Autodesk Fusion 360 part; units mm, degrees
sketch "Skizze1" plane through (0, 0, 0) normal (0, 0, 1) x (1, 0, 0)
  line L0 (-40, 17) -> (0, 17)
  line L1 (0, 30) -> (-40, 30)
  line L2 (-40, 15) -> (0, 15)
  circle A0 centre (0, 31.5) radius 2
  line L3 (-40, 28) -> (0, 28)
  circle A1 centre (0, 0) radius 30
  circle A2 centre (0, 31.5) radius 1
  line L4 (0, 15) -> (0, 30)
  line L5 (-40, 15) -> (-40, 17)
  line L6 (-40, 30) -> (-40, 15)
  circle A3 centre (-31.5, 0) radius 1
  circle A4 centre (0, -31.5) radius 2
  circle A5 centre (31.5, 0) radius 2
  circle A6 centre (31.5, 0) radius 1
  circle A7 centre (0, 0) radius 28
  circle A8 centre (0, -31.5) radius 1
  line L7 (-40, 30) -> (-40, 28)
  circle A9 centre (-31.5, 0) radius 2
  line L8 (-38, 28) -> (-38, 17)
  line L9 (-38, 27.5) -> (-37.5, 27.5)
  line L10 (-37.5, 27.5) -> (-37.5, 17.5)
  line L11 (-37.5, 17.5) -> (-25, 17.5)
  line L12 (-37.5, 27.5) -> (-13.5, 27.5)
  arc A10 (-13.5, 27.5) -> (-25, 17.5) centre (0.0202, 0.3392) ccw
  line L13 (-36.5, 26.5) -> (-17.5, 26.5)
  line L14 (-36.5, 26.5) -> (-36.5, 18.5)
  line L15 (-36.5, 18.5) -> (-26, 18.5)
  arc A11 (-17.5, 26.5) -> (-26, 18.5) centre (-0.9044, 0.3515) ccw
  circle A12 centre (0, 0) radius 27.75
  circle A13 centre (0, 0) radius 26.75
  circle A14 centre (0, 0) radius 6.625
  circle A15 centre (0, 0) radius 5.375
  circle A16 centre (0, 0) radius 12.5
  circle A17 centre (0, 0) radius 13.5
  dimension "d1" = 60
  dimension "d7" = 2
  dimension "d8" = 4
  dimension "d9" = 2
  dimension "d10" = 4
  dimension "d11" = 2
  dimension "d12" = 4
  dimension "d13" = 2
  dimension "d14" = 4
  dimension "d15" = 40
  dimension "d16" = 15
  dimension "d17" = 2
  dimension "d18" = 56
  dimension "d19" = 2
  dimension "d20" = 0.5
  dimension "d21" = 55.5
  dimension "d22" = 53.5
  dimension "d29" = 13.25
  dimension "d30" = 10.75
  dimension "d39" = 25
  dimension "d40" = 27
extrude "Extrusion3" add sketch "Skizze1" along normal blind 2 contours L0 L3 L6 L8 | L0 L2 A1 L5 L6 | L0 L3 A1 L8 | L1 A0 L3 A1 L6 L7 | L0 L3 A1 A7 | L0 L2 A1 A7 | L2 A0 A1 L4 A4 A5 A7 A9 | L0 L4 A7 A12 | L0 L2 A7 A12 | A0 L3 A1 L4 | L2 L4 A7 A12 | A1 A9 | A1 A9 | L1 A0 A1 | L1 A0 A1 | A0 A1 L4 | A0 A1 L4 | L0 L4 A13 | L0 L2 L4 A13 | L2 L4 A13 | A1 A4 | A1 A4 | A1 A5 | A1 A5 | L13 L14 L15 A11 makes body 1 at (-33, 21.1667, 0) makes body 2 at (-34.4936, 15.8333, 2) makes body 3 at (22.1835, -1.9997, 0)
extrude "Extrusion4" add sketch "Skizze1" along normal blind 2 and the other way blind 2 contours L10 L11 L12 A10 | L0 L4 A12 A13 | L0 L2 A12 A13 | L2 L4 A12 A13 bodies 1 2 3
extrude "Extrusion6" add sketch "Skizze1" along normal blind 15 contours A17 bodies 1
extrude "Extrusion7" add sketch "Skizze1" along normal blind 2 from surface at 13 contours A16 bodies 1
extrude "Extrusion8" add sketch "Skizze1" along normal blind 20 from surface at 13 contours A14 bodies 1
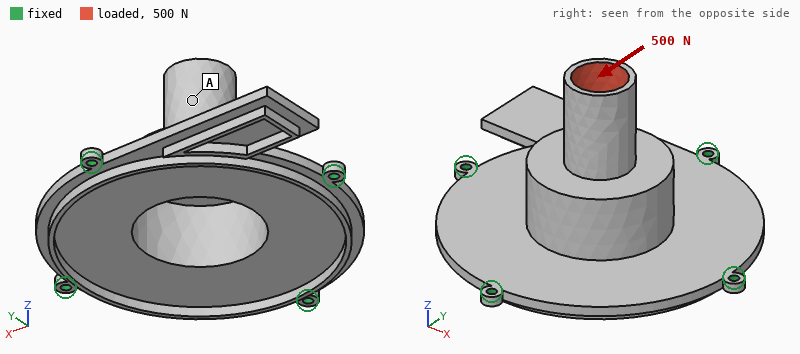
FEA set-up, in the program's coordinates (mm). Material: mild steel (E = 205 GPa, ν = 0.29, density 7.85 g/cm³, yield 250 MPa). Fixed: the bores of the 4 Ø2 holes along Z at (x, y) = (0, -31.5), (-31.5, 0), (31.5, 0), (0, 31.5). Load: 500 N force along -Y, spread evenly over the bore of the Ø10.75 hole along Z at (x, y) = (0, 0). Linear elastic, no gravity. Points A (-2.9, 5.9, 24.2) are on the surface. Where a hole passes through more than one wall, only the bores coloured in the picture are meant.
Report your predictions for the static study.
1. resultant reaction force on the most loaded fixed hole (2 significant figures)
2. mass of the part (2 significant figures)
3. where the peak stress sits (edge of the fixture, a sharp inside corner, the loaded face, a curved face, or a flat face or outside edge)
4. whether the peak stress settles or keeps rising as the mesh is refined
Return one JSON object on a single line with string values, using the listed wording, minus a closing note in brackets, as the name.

{"resultant reaction force on the most loaded fixed hole": "250 N", "mass of the part": "67 g", "where the peak stress sits": "edge of the fixture", "whether the peak stress settles or keeps rising as the mesh is refined": "keeps rising"}
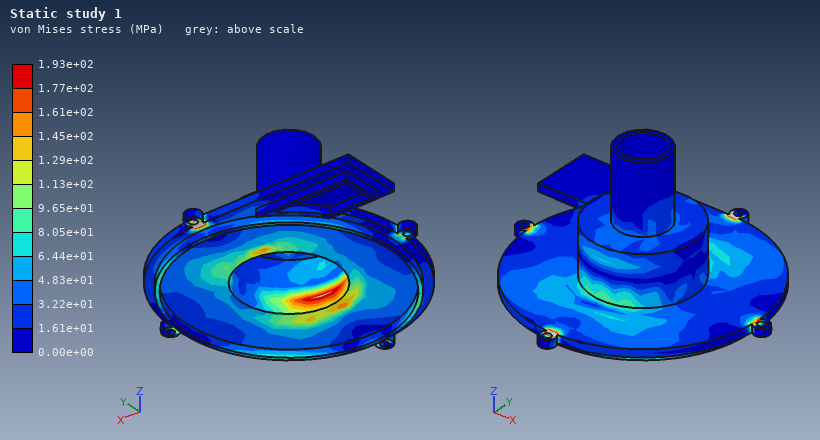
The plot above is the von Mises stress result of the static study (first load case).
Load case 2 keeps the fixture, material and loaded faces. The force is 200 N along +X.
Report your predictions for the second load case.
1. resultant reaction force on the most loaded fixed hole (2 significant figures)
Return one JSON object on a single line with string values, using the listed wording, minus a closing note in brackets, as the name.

{"resultant reaction force on the most loaded fixed hole": "100 N"}
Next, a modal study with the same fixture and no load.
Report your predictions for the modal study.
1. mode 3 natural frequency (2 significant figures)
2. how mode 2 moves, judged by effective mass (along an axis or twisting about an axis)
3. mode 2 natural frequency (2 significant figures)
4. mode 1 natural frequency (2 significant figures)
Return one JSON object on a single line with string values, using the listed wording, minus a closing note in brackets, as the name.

{"mode 3 natural frequency": "3200 Hz", "how mode 2 moves, judged by effective mass": "along Z", "mode 2 natural frequency": "2900 Hz", "mode 1 natural frequency": "2000 Hz"}
